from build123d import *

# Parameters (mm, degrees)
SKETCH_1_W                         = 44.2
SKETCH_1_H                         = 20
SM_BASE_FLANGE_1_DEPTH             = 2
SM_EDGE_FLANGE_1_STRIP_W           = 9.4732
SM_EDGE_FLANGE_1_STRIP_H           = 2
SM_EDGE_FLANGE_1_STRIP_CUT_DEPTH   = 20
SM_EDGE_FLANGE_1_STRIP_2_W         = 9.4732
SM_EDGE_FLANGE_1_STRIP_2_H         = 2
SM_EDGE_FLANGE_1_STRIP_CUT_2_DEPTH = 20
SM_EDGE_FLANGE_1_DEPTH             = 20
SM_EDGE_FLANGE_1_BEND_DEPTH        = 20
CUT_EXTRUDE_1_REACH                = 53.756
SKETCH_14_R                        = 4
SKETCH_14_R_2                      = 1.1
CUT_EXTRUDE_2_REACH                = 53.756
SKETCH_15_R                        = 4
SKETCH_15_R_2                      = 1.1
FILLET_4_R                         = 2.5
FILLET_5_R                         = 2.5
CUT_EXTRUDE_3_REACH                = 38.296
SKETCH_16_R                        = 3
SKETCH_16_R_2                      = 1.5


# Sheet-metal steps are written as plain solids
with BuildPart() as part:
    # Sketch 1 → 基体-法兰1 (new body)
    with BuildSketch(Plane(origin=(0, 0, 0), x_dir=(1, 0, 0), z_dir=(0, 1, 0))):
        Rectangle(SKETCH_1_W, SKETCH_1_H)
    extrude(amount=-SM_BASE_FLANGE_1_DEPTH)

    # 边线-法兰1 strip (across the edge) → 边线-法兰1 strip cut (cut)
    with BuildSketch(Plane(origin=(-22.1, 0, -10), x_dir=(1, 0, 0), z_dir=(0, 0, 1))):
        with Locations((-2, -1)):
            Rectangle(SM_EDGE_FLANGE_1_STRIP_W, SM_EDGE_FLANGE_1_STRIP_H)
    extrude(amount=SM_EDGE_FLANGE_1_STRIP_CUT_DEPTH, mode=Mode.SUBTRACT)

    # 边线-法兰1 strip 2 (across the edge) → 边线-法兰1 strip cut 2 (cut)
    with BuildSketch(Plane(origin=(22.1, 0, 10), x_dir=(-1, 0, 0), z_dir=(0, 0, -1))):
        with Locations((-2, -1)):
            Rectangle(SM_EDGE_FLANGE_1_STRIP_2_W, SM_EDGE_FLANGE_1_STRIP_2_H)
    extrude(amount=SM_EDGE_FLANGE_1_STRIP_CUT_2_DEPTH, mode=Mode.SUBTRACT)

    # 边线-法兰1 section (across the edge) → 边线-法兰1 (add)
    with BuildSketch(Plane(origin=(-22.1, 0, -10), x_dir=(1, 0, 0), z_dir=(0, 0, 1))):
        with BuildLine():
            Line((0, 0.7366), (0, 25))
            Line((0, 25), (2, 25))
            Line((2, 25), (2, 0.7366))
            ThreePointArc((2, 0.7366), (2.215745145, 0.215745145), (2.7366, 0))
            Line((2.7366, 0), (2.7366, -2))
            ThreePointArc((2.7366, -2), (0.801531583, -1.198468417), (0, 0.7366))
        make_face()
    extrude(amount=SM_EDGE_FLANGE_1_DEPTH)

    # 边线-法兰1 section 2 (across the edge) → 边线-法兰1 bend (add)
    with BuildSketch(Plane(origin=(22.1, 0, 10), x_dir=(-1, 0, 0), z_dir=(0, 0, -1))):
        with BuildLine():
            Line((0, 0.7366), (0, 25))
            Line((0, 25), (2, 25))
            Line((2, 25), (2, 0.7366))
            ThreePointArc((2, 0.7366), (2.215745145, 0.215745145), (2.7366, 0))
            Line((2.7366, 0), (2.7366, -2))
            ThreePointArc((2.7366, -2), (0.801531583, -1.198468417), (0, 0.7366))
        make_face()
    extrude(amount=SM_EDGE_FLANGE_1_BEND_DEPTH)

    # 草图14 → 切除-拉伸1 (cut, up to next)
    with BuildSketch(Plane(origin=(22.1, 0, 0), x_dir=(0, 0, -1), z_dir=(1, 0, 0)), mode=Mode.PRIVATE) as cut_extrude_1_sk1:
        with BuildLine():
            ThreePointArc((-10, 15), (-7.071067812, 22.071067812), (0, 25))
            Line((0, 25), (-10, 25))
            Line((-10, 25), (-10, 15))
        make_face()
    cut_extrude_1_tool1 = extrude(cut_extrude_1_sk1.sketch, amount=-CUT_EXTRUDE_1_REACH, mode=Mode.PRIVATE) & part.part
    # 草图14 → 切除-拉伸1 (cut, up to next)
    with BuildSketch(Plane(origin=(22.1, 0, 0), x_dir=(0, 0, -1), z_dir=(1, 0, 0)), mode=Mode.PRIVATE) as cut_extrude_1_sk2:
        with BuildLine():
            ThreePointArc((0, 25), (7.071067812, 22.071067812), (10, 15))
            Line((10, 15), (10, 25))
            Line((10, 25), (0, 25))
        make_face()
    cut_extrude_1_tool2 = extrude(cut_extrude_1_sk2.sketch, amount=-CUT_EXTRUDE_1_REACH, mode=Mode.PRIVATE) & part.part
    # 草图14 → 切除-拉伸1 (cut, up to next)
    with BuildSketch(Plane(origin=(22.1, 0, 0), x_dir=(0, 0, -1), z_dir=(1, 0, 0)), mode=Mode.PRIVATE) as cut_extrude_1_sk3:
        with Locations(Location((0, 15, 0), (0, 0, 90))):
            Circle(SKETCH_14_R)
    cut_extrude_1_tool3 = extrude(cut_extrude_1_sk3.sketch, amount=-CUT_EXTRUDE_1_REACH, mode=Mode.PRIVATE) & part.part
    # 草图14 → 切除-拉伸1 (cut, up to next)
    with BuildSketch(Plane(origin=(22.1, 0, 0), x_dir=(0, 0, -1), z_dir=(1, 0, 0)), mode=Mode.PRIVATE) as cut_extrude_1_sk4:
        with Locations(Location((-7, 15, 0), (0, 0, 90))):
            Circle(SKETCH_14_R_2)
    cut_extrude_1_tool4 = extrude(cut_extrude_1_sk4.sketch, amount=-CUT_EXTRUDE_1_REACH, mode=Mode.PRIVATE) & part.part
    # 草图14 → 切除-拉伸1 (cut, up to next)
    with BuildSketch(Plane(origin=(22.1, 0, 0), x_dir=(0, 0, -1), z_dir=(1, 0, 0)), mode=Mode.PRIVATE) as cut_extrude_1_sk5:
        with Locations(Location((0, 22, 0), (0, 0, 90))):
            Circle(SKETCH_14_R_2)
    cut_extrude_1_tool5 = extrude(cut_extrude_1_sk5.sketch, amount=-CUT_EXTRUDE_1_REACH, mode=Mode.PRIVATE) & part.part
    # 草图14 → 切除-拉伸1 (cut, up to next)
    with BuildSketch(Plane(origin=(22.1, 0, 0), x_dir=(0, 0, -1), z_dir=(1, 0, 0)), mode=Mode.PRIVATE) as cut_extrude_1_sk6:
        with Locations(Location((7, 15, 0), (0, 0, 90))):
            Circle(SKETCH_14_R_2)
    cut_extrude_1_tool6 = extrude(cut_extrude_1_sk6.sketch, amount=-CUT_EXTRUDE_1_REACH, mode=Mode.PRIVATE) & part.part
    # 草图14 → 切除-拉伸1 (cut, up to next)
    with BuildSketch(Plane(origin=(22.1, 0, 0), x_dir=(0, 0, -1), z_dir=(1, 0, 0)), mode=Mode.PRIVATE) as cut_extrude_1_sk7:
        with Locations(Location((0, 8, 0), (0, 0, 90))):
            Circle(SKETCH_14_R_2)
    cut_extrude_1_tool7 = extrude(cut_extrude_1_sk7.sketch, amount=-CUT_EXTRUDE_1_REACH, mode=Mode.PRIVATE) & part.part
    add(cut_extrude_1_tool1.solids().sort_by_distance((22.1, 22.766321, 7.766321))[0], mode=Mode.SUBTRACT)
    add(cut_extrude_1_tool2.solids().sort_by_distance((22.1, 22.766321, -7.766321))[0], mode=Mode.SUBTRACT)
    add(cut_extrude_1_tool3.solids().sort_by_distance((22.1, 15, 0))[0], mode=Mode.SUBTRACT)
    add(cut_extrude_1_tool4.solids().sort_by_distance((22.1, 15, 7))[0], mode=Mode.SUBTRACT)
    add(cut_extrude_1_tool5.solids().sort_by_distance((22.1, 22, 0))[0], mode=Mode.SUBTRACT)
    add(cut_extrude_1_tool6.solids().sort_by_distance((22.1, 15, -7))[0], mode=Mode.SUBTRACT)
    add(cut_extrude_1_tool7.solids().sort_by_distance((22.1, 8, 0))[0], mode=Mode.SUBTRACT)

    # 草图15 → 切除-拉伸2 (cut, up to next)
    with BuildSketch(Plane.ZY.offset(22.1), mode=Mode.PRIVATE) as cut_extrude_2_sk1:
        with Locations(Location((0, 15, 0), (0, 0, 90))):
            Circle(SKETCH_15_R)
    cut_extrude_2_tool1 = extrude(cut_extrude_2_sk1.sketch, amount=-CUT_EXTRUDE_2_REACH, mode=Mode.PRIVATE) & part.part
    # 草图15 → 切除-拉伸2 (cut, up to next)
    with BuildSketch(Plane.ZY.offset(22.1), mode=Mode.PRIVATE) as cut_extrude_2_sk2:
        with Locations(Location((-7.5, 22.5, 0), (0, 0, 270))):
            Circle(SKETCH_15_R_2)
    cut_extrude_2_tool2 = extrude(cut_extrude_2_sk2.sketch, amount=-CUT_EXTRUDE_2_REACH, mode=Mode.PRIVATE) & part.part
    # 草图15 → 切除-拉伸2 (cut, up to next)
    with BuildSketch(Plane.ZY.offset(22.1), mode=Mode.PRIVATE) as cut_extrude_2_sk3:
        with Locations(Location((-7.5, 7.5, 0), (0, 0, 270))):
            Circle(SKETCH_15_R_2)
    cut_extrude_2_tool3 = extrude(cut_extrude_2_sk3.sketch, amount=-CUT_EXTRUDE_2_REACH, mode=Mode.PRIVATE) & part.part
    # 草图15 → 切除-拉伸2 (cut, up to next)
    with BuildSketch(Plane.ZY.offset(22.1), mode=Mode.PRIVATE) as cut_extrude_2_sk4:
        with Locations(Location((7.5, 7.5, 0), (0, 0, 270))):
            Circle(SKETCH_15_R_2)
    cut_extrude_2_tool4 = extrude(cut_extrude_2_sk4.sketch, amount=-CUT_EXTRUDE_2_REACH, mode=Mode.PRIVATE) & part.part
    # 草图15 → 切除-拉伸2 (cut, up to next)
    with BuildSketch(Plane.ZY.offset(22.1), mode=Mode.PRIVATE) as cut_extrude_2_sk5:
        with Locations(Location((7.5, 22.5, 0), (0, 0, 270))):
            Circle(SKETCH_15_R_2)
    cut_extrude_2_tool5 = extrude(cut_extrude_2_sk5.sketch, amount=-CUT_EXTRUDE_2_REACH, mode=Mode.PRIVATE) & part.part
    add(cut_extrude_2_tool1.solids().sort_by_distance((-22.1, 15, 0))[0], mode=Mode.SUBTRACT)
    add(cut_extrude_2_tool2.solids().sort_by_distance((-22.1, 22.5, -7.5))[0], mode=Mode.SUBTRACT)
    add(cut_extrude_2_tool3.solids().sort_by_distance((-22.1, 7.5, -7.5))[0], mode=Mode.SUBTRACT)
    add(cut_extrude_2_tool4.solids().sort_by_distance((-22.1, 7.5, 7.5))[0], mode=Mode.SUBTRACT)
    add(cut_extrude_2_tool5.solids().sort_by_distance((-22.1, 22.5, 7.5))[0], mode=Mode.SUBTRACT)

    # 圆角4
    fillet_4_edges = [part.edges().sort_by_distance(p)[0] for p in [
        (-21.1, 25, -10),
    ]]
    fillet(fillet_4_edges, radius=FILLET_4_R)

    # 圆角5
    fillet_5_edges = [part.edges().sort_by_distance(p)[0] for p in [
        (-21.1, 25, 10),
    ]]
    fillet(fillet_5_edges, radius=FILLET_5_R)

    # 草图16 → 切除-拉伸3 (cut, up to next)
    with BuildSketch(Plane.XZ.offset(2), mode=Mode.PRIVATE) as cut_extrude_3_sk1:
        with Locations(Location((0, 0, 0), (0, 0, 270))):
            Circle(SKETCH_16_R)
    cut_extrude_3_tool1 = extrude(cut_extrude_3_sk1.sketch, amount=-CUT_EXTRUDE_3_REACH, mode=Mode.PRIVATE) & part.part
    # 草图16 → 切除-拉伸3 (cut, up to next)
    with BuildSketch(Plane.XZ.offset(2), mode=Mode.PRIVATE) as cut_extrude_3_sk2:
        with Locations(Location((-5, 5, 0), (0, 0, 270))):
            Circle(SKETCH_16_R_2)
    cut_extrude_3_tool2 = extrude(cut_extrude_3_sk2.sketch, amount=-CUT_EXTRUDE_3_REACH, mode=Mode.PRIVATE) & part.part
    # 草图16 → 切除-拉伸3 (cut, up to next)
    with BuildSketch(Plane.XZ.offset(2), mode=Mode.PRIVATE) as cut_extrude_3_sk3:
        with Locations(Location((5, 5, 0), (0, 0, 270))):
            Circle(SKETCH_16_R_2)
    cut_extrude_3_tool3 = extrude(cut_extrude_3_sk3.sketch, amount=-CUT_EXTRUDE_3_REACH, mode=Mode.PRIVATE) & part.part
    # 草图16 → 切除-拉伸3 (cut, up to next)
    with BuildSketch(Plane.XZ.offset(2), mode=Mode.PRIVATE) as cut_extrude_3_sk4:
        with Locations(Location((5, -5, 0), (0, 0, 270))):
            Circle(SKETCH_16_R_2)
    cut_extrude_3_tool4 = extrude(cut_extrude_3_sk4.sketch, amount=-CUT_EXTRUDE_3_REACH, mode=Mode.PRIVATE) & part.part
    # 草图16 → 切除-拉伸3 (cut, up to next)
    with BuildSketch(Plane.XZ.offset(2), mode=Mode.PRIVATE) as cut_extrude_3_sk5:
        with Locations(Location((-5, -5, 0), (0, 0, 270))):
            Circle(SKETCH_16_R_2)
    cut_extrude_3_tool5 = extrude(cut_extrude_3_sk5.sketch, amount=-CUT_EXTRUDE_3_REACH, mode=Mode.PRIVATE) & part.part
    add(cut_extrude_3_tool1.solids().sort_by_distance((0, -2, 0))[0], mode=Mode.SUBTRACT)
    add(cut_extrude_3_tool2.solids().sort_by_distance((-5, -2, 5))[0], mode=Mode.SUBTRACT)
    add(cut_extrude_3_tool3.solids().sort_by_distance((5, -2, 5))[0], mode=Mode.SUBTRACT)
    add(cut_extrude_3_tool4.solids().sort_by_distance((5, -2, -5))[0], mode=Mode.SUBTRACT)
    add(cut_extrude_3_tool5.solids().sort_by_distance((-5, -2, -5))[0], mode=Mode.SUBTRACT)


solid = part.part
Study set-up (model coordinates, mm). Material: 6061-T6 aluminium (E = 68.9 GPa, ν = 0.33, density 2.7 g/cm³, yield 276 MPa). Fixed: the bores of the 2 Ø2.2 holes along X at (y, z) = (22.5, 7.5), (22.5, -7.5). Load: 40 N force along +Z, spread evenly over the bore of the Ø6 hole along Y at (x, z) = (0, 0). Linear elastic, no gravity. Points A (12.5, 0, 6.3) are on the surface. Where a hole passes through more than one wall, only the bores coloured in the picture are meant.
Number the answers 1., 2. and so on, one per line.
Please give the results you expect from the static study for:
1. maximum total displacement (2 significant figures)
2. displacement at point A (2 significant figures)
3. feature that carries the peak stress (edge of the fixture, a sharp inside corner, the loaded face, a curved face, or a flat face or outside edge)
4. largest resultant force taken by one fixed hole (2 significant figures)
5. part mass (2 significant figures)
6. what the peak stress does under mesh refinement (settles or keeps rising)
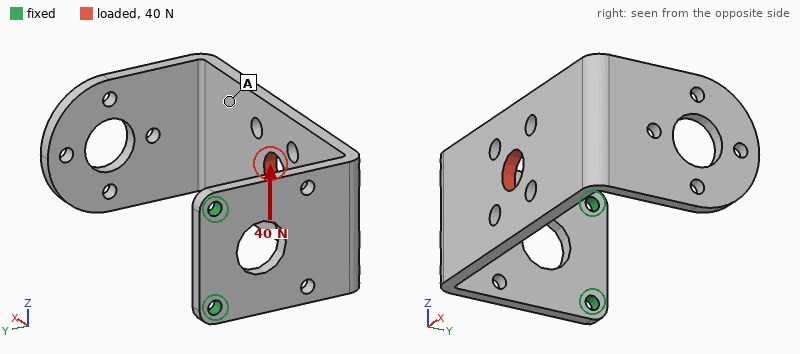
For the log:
1. 0.58 mm
2. 0.42 mm
3. edge of the fixture
4. 79 N
5. 8.8 g
6. keeps rising
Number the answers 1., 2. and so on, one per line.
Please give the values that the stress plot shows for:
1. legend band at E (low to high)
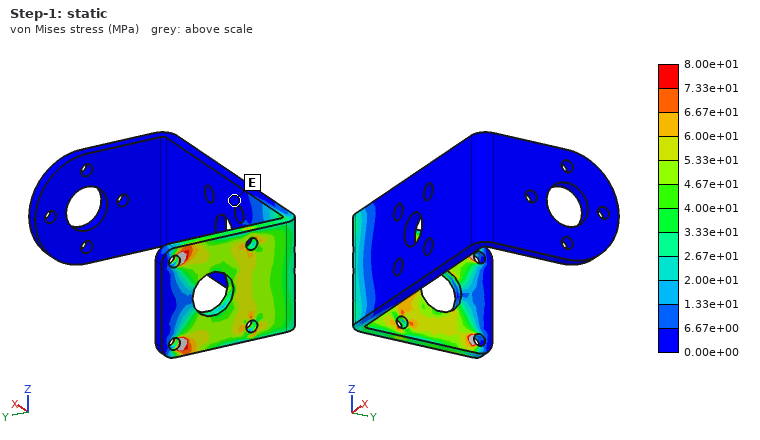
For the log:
1. 0.00e+00 to 6.67e+00 MPa
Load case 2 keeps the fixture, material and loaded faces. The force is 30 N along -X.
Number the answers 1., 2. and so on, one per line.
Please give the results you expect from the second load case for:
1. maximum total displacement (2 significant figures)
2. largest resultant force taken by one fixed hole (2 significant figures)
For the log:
1. 0.55 mm
2. 15 N
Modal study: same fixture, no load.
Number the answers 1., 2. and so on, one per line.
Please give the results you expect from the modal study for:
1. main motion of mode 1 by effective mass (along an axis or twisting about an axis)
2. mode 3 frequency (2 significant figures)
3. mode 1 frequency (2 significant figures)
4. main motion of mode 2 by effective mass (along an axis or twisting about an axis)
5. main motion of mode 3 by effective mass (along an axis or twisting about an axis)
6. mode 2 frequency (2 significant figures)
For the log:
1. along Y
2. 920 Hz
3. 280 Hz
4. along Z
5. along X
6. 480 Hz
